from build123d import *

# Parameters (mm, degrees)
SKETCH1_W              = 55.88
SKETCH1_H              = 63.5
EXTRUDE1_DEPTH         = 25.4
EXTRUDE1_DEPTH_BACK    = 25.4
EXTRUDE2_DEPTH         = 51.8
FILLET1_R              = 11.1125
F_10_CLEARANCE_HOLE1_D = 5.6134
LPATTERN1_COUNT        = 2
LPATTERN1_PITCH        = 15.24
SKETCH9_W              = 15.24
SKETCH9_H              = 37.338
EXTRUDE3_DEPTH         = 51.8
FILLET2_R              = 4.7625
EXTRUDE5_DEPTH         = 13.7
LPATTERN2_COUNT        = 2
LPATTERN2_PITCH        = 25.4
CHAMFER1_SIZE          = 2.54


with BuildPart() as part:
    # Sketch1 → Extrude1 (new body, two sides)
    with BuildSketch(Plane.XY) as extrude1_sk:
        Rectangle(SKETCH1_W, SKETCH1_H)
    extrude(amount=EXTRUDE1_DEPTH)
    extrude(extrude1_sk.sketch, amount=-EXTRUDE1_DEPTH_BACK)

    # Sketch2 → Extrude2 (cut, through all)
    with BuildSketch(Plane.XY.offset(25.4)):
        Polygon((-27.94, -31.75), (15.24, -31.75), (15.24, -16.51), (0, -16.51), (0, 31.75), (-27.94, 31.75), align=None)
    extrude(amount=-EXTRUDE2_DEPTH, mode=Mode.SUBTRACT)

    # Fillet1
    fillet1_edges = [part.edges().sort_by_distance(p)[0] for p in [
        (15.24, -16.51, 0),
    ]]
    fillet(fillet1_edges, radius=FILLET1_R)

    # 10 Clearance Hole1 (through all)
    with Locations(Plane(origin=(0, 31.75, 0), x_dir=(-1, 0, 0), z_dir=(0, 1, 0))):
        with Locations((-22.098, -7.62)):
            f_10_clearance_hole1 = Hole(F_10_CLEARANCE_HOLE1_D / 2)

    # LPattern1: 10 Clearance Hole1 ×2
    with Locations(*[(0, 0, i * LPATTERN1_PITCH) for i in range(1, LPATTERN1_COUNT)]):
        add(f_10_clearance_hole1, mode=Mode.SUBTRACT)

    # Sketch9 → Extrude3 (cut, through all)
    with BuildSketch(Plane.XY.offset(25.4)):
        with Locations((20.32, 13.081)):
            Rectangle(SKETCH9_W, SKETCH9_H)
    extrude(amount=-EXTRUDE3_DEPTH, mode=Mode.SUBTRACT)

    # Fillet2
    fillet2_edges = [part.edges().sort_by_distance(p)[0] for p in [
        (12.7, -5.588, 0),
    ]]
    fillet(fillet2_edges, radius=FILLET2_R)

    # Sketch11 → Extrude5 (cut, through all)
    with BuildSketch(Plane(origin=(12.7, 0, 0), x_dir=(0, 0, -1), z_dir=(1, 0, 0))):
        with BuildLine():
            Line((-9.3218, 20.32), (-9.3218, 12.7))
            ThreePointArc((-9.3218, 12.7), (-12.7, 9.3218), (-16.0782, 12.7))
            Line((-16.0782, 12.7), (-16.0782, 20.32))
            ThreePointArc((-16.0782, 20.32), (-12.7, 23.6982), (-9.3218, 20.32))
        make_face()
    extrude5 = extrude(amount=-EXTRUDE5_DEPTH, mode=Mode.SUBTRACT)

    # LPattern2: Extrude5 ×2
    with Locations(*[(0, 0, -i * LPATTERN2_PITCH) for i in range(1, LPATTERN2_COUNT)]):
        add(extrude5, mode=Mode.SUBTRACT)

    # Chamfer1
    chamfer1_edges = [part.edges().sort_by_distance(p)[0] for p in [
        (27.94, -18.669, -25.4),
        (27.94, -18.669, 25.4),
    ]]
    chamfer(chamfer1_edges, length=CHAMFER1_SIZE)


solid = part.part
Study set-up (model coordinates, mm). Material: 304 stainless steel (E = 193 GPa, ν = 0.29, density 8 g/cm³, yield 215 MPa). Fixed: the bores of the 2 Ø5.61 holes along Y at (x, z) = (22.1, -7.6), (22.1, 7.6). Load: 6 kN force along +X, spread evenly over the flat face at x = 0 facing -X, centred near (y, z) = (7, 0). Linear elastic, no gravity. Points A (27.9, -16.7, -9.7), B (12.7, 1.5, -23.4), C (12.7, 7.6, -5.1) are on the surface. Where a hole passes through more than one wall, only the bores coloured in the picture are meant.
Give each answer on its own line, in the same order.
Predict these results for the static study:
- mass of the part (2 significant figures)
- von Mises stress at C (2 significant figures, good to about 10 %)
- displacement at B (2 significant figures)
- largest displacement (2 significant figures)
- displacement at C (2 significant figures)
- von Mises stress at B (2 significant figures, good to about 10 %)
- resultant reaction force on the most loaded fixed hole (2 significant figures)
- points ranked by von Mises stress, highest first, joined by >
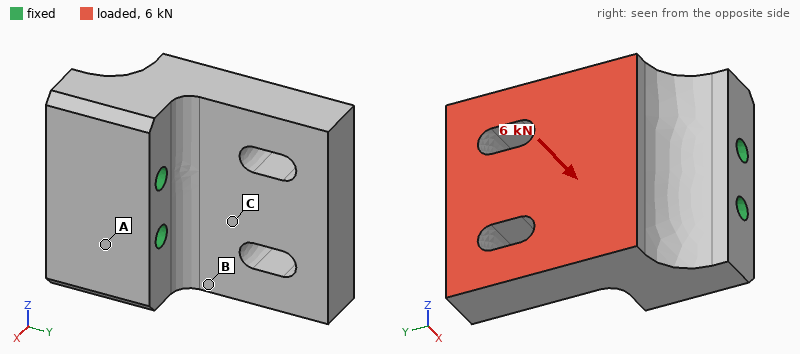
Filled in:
380 g
27 MPa
11 µm
52 µm
18 µm
42 MPa
3.0 kN
B > C > A
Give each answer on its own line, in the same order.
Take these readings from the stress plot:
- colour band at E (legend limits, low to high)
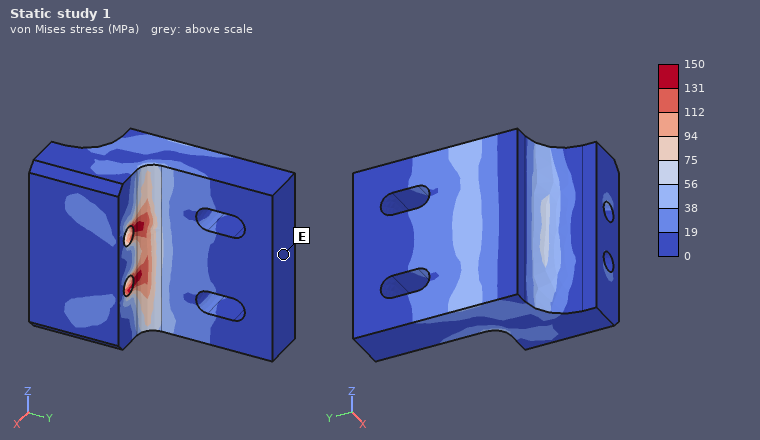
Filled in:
0 to 19 MPa
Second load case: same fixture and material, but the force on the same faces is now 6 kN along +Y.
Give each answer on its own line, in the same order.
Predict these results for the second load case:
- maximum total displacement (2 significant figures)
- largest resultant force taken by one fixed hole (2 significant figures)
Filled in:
34 µm
3.0 kN
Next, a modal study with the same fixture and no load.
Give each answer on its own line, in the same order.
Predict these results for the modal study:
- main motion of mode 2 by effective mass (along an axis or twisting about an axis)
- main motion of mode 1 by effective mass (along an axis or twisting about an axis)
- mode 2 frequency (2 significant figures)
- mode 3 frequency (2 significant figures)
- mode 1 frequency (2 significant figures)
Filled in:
along Z
along X
6900 Hz
8400 Hz
4300 Hz
